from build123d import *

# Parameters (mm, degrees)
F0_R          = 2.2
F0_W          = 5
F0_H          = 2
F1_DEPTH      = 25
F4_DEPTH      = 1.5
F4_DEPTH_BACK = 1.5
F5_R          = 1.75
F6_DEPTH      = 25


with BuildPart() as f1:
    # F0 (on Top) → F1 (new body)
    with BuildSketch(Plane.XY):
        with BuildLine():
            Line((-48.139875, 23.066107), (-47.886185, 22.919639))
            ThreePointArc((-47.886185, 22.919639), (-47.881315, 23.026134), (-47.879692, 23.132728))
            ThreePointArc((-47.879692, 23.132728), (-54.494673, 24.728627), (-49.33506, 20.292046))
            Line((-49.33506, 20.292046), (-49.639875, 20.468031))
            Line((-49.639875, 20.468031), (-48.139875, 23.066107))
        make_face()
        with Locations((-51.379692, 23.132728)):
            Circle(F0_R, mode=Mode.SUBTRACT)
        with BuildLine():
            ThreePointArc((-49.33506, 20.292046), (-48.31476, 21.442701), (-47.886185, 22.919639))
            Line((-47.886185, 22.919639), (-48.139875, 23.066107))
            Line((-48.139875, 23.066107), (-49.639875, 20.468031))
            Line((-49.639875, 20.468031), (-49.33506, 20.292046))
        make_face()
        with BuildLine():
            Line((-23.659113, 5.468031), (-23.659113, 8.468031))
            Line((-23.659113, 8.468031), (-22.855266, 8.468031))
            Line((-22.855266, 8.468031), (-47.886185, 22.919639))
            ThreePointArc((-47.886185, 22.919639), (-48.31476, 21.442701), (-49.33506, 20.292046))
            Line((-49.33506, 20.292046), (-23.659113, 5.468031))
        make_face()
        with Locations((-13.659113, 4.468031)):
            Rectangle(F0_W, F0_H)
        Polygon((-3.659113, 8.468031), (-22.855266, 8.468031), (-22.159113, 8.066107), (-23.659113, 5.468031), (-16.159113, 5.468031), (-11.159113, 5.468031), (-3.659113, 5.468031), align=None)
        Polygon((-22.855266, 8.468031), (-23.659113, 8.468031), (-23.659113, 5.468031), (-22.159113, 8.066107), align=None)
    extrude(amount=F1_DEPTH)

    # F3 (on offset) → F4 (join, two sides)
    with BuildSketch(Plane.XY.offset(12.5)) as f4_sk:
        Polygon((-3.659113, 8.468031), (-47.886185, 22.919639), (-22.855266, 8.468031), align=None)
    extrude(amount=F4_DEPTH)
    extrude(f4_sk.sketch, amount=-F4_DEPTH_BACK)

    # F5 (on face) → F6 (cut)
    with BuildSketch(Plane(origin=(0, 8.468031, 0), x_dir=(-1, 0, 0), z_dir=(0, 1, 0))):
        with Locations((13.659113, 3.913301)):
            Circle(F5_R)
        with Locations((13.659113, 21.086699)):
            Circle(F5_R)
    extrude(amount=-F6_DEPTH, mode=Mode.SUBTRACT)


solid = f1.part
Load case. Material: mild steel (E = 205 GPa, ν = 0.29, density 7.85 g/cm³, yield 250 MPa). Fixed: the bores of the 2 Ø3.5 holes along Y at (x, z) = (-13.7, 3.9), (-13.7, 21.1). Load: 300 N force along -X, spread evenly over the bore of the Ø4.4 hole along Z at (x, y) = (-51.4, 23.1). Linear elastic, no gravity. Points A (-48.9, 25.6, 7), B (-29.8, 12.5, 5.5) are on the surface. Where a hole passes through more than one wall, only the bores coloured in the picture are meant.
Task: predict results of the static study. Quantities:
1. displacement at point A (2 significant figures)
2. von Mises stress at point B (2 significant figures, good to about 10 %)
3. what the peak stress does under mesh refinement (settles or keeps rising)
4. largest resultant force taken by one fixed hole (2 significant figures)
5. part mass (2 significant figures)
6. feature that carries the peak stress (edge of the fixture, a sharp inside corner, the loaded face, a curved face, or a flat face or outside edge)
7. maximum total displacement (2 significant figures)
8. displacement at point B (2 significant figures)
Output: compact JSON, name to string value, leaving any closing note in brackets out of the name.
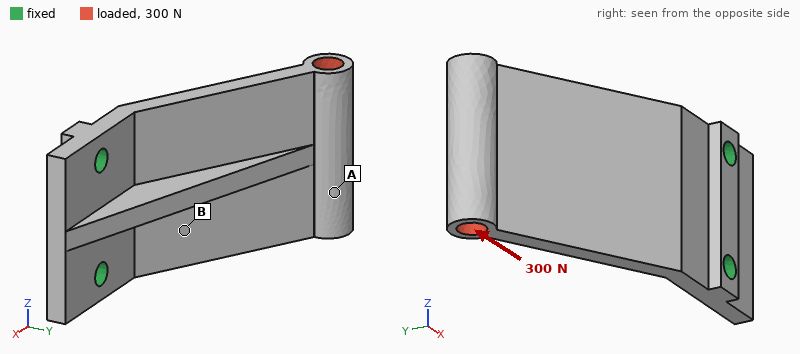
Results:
{"displacement at point A": "0.088 mm", "von Mises stress at point B": "20 MPa", "what the peak stress does under mesh refinement": "keeps rising", "largest resultant force taken by one fixed hole": "150 N", "part mass": "38 g", "feature that carries the peak stress": "edge of the fixture", "maximum total displacement": "0.10 mm", "displacement at point B": "0.021 mm"}
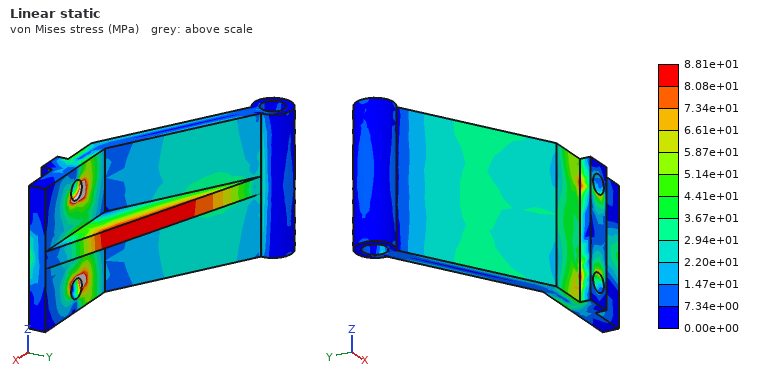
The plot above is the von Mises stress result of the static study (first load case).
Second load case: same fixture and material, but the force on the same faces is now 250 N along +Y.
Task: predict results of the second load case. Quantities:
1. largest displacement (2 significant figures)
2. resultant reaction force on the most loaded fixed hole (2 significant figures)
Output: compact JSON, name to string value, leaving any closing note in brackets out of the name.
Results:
{"largest displacement": "0.17 mm", "resultant reaction force on the most loaded fixed hole": "140 N"}
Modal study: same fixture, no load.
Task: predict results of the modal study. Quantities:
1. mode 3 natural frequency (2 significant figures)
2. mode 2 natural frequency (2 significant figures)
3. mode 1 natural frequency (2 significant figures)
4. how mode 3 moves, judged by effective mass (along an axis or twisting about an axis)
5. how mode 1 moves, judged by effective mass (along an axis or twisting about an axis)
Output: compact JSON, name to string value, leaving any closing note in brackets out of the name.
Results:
{"mode 3 natural frequency": "7100 Hz", "mode 2 natural frequency": "4900 Hz", "mode 1 natural frequency": "2000 Hz", "how mode 3 moves, judged by effective mass": "along Z", "how mode 1 moves, judged by effective mass": "along Y"}
